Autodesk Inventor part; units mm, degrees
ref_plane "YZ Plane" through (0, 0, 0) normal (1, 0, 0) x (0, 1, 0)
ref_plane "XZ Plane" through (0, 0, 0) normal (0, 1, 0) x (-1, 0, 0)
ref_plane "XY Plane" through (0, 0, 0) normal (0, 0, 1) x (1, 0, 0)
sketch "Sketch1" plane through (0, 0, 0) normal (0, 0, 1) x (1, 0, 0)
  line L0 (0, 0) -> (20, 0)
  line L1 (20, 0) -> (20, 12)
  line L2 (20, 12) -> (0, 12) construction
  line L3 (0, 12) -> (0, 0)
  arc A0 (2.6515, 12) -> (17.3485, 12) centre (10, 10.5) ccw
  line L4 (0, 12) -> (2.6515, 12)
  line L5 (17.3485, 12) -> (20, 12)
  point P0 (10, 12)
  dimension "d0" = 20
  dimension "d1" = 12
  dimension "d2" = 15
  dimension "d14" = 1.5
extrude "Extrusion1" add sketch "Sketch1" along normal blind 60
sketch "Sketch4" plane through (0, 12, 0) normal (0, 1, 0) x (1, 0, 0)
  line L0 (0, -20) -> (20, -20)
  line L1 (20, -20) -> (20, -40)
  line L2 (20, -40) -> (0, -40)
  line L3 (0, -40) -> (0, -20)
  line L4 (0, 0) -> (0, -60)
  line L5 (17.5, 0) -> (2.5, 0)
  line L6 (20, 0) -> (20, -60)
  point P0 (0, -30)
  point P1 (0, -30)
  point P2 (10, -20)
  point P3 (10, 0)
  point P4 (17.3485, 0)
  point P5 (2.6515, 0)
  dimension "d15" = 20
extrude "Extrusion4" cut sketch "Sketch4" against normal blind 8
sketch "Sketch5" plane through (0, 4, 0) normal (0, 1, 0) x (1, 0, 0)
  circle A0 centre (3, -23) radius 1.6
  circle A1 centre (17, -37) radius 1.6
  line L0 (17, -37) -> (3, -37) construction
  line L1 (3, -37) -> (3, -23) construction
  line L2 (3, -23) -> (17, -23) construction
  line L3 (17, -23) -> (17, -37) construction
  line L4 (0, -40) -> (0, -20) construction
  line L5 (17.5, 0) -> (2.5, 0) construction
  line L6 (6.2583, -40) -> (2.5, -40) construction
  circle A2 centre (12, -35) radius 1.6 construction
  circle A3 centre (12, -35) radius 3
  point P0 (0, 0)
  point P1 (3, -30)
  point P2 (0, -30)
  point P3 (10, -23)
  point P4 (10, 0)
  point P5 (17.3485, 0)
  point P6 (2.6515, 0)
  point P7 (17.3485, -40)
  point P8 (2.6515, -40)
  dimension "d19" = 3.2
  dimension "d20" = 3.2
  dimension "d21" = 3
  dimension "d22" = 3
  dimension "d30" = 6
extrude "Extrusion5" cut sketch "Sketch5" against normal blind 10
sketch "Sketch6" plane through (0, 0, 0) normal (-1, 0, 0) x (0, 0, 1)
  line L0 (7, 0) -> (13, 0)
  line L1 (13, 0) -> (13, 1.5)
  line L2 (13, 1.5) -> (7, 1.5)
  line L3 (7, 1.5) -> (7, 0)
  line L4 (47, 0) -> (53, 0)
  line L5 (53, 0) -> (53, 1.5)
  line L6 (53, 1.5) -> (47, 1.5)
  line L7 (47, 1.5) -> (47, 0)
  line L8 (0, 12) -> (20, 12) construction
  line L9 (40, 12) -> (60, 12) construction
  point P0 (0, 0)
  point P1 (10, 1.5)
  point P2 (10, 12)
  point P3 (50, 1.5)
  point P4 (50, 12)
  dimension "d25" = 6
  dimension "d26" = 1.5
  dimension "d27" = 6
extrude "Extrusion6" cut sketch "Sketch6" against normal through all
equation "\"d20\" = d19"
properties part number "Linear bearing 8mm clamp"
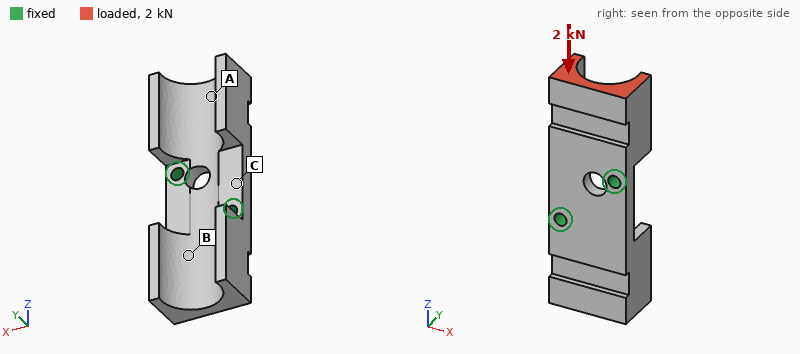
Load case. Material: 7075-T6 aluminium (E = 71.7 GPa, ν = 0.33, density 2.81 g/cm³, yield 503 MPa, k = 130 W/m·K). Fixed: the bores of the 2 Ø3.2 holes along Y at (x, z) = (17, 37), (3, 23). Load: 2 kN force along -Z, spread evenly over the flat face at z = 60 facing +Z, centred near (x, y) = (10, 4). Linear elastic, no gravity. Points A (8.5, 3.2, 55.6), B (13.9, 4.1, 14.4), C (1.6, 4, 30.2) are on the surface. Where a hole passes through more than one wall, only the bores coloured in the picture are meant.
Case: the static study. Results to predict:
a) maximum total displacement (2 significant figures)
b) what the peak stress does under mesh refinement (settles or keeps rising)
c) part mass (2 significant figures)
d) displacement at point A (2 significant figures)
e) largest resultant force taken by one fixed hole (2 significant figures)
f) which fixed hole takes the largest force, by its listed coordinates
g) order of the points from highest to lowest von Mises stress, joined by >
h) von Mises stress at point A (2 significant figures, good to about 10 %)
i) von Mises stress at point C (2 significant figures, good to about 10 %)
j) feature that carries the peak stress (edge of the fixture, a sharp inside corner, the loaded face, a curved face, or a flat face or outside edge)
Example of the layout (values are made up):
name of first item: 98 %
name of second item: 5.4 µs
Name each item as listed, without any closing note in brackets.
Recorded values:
maximum total displacement: 0.13 mm
what the peak stress does under mesh refinement: keeps rising
part mass: 17 g
displacement at point A: 0.083 mm
largest resultant force taken by one fixed hole: 1.1 kN
which fixed hole takes the largest force, by its listed coordinates: (17, 37)
order of the points from highest to lowest von Mises stress, joined by >: C > A > B
von Mises stress at point A: 22 MPa
von Mises stress at point C: 60 MPa
feature that carries the peak stress: edge of the fixture
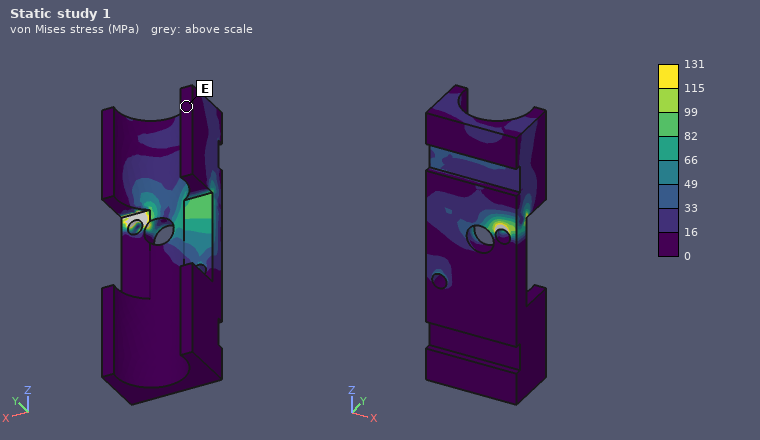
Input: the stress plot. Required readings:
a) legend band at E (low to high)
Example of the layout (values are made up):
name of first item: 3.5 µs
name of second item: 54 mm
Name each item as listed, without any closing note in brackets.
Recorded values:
legend band at E: 0 to 16 MPa
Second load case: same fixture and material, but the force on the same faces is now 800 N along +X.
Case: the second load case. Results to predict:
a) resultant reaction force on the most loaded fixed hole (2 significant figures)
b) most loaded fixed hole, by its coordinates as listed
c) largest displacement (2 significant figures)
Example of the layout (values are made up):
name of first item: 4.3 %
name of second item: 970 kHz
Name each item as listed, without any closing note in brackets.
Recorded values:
resultant reaction force on the most loaded fixed hole: 1.4 kN
most loaded fixed hole, by its coordinates as listed: (17, 37)
largest displacement: 91 µm
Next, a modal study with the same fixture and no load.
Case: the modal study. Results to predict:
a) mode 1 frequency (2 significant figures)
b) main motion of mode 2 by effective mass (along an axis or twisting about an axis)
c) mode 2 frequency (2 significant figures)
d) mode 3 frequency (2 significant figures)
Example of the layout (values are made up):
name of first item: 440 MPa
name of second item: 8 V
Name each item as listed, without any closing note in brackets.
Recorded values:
mode 1 frequency: 3800 Hz
main motion of mode 2 by effective mass: along Y
mode 2 frequency: 4000 Hz
mode 3 frequency: 7600 Hz
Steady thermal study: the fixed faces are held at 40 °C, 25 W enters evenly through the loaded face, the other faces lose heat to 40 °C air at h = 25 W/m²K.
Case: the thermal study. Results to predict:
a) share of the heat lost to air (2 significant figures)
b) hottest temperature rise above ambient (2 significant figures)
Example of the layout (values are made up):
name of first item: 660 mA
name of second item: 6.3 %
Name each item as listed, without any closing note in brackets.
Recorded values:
share of the heat lost to air: 6.5 %
hottest temperature rise above ambient: 54 K
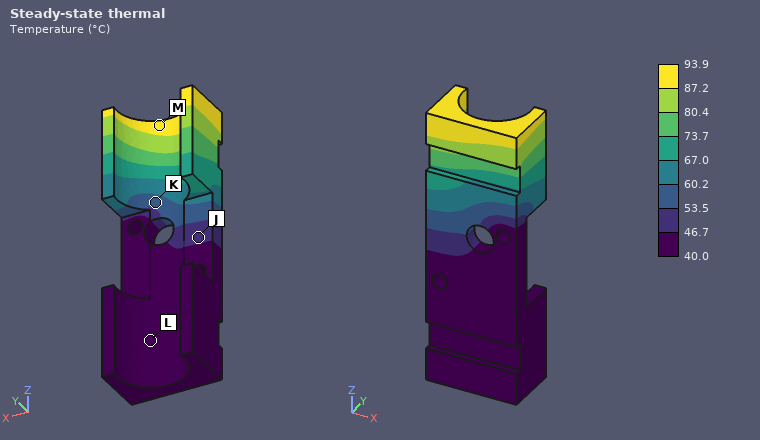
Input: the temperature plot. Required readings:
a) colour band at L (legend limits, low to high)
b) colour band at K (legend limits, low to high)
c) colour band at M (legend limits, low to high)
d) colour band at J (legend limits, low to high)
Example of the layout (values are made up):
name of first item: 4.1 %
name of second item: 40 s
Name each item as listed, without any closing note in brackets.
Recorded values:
colour band at L: 40.0 to 46.7 °C
colour band at K: 53.5 to 60.2 °C
colour band at M: 87.2 to 93.9 °C
colour band at J: 46.7 to 53.5 °C
